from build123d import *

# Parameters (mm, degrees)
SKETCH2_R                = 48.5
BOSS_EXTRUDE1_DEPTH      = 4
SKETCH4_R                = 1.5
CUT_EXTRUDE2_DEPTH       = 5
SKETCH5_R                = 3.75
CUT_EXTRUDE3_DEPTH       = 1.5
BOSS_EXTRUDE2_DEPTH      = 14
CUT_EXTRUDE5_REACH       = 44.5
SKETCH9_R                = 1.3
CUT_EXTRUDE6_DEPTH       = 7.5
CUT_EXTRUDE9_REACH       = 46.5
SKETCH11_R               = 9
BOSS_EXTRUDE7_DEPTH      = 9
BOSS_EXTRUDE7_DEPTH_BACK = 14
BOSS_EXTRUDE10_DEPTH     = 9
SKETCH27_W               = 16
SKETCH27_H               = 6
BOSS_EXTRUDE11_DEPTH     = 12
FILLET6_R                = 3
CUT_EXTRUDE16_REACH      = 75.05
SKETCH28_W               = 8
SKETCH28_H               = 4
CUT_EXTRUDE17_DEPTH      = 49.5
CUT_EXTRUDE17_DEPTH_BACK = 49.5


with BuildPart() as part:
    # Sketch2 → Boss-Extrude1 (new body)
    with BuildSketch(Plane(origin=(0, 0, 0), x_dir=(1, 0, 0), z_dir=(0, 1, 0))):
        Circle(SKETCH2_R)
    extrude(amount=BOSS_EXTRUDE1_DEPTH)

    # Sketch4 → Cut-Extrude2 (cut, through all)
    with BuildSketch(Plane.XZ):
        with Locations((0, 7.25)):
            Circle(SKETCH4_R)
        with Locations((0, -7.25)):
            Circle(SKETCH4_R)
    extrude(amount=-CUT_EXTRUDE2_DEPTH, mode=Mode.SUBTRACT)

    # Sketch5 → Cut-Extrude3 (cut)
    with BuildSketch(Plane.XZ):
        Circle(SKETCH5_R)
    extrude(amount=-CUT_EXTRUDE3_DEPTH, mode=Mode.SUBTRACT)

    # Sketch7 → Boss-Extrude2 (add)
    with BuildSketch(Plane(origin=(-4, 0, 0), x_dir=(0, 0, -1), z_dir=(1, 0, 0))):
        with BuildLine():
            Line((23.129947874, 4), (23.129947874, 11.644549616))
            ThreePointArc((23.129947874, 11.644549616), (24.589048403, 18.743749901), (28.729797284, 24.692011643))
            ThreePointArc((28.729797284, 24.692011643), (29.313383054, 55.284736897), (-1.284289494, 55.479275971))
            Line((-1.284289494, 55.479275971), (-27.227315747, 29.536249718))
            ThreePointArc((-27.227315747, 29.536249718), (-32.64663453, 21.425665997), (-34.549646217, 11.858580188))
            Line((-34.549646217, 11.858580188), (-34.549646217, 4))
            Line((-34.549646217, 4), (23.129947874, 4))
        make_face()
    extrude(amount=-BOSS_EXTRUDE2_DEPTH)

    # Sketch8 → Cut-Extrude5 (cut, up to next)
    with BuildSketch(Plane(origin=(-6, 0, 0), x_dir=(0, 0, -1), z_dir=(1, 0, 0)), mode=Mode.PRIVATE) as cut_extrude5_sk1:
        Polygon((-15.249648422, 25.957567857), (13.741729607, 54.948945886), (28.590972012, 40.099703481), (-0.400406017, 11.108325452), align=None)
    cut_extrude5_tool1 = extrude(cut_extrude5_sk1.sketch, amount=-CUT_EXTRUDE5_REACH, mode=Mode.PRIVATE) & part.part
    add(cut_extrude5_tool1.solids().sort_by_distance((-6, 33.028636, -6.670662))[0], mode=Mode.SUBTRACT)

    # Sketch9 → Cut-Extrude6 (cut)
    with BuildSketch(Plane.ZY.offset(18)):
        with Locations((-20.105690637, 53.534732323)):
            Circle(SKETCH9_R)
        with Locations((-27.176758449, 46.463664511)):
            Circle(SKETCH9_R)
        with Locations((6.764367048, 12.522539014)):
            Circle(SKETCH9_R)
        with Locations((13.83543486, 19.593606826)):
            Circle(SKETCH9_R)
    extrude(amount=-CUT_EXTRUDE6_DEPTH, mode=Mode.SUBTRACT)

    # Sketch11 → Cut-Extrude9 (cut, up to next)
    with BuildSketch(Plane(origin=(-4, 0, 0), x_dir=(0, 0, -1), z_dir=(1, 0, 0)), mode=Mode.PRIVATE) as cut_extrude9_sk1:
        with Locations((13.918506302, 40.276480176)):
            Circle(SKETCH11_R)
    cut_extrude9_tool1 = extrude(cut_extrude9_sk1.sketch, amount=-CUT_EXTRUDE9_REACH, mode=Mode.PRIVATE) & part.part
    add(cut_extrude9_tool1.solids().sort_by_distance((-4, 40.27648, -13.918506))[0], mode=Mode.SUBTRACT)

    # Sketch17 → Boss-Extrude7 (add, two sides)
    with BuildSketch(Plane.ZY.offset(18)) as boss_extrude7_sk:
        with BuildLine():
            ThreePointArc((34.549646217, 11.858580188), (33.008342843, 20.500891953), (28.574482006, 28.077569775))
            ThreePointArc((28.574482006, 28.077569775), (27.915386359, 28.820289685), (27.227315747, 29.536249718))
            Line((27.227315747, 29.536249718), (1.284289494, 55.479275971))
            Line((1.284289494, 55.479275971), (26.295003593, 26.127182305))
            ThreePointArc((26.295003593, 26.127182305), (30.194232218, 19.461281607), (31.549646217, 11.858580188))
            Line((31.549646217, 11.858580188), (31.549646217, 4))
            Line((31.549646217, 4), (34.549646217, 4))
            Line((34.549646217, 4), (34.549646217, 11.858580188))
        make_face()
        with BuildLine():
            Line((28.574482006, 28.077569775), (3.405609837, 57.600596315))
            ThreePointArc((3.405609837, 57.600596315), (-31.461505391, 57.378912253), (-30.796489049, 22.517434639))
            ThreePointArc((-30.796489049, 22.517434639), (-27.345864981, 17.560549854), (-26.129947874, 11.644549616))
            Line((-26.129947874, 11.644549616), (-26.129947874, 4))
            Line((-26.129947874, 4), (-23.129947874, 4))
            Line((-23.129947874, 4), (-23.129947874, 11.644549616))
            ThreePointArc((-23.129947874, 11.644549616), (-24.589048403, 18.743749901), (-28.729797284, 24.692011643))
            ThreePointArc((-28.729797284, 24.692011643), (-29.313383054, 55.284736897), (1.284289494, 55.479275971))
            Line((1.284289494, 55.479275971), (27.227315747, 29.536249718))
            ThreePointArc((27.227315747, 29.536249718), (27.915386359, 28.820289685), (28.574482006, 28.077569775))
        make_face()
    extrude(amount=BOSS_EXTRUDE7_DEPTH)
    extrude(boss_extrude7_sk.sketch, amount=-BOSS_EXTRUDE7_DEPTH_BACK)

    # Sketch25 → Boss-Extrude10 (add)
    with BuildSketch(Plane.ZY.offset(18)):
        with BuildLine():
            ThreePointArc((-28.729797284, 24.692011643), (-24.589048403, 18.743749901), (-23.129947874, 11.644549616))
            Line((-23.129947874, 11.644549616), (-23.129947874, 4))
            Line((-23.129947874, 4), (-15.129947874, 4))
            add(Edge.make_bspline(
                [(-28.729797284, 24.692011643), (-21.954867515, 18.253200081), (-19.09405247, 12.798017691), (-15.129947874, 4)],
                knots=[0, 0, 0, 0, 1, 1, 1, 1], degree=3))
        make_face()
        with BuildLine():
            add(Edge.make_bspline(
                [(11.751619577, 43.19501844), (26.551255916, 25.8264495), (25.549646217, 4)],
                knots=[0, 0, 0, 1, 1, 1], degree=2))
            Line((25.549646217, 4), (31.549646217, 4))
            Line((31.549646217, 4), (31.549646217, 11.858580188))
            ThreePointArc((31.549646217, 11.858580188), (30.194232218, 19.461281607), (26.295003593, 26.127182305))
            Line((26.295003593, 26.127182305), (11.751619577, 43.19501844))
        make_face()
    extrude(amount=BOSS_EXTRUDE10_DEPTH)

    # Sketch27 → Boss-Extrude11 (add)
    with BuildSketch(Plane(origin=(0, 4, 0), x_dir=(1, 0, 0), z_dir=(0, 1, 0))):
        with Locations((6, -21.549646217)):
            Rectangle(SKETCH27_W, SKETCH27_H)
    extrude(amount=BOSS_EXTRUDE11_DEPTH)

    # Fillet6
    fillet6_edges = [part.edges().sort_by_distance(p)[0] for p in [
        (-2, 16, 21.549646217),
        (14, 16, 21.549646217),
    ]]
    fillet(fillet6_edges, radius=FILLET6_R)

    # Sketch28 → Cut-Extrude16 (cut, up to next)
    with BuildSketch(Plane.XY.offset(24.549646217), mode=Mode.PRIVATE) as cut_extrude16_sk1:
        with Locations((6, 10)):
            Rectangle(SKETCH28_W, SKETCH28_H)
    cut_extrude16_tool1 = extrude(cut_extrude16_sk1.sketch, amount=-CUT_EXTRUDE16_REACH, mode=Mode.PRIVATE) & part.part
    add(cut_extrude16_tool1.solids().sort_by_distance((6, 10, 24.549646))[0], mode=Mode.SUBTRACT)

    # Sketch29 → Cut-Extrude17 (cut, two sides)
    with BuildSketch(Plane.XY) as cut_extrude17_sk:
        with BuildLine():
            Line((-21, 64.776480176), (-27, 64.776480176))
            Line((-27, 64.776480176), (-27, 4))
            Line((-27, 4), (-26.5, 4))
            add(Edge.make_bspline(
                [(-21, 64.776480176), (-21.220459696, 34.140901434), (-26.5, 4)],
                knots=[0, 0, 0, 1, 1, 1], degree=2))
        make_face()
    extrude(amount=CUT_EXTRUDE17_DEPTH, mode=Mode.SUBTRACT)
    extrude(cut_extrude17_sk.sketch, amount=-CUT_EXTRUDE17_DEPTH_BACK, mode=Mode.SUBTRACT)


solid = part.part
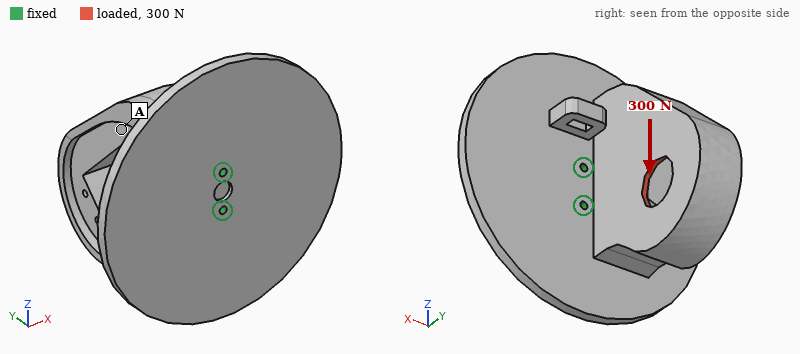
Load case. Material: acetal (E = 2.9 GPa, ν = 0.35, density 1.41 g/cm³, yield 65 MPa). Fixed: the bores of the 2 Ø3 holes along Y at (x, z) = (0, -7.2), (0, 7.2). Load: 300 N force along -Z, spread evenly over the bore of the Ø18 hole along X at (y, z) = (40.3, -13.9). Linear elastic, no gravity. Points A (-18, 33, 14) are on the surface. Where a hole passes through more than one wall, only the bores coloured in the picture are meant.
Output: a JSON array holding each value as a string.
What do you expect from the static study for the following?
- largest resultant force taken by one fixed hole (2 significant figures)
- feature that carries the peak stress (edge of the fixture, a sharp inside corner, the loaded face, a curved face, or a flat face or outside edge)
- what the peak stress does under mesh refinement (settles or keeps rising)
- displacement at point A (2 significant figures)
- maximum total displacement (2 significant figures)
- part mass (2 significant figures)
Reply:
["630 N", "edge of the fixture", "keeps rising", "0.60 mm", "1.2 mm", "96 g"]
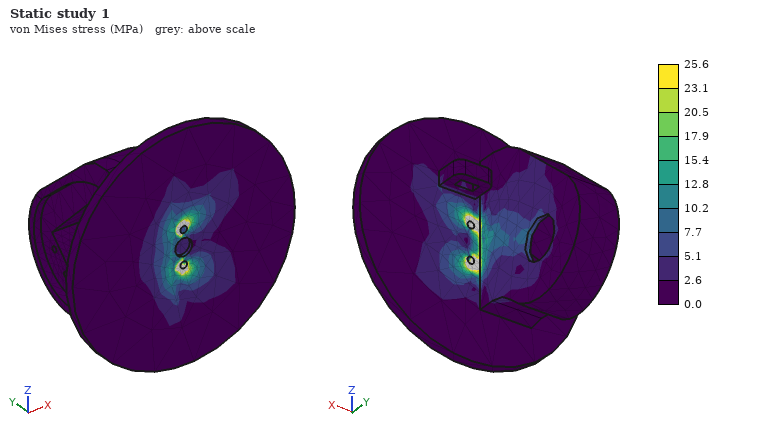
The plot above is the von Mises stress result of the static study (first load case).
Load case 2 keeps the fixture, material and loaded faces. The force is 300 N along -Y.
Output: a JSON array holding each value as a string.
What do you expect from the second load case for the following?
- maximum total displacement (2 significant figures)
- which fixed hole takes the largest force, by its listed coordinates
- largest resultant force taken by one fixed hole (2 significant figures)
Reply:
["0.65 mm", "(0, -7.2)", "370 N"]
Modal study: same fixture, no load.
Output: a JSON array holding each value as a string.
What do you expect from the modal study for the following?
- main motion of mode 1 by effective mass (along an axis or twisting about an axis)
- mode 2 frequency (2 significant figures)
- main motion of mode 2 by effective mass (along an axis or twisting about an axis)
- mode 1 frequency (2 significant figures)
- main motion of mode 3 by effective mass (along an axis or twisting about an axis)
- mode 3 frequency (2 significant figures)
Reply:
["along X", "400 Hz", "along Z", "180 Hz", "along Y", "490 Hz"]
